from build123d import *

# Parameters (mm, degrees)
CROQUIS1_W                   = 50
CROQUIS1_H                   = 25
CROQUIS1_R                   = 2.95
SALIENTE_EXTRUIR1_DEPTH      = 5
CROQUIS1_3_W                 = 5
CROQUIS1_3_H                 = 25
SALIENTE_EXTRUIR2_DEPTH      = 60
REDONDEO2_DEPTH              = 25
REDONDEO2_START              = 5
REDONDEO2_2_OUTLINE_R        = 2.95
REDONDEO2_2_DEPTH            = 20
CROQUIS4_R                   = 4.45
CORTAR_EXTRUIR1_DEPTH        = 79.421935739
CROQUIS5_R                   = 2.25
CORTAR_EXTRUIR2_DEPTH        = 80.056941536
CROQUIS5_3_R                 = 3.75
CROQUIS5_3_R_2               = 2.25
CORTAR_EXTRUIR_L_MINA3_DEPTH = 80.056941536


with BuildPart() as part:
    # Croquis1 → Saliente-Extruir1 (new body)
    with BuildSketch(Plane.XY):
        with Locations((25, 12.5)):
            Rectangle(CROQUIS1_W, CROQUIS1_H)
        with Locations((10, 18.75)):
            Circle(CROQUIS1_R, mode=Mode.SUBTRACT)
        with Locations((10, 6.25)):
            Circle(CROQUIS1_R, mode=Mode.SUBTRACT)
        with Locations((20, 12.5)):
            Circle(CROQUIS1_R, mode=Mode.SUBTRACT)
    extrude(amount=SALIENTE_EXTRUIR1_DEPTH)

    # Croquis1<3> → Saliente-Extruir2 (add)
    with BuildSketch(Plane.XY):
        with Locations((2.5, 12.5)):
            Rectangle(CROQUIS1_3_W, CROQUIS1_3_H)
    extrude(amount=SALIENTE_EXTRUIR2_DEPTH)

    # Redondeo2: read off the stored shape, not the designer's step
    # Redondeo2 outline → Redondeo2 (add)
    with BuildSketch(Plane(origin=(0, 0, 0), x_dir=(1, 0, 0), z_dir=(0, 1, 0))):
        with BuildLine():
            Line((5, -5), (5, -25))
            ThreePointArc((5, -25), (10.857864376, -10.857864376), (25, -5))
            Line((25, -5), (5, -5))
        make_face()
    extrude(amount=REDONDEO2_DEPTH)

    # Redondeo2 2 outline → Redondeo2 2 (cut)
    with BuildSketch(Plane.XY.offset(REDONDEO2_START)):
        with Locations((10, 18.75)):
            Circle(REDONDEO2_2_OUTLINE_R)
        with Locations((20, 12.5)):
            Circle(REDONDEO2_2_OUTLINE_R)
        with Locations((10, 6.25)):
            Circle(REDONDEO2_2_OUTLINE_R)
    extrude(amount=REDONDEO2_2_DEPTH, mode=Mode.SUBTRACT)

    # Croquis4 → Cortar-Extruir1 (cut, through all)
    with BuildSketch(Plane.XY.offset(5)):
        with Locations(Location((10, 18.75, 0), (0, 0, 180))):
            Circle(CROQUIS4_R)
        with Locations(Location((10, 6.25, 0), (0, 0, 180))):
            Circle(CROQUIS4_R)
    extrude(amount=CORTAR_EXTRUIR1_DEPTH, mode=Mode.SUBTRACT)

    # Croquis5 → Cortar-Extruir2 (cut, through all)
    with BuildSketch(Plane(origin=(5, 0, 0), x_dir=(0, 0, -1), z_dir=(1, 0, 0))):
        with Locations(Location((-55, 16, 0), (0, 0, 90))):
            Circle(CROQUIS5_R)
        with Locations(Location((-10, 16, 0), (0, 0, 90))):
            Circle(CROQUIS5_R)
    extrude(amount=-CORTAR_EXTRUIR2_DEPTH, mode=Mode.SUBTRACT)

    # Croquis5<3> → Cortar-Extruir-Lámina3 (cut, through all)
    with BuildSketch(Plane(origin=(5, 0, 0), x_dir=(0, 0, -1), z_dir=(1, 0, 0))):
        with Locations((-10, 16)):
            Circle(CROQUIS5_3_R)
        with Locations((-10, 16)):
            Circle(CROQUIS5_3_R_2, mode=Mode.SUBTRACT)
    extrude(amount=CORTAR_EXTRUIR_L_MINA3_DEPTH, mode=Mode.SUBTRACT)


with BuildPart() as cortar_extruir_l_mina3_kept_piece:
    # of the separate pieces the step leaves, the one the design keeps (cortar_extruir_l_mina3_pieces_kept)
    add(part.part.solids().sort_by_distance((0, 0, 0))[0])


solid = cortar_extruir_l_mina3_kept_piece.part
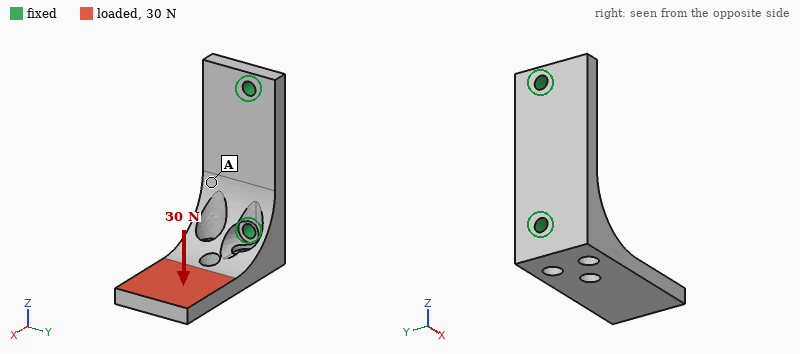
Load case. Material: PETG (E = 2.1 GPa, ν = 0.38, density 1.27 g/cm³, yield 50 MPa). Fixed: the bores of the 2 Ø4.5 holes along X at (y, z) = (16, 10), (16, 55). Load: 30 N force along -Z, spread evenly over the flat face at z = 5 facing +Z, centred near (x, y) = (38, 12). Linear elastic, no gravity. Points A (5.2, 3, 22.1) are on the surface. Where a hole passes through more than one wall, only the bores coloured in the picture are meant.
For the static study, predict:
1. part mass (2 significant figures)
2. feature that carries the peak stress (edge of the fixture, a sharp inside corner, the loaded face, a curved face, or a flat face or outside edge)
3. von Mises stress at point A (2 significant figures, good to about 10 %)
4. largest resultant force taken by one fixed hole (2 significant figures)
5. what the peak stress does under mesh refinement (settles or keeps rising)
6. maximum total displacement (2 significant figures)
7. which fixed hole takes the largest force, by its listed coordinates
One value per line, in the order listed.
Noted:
17 g
edge of the fixture
2.0 MPa
21 N
keeps rising
0.79 mm
(16, 10)
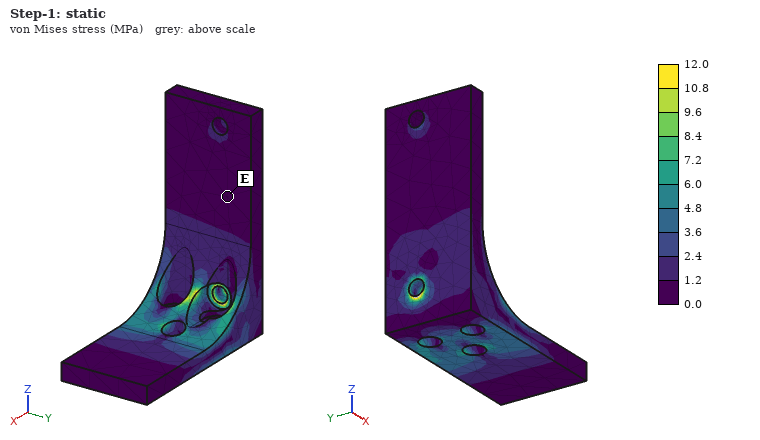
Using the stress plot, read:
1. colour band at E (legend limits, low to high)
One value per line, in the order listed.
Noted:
0.0 to 1.2 MPa
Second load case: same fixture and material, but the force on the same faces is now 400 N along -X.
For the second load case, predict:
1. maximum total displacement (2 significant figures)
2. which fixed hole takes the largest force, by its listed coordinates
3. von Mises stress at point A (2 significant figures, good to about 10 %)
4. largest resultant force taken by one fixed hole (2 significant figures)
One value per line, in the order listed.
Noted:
0.70 mm
(16, 10)
3.4 MPa
410 N
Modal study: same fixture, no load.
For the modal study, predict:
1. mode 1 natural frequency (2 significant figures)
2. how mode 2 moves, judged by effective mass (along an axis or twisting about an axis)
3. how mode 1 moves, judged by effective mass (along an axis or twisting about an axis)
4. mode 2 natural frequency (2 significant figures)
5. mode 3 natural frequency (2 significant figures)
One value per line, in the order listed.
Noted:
580 Hz
along Y
along Z
780 Hz
2000 Hz
